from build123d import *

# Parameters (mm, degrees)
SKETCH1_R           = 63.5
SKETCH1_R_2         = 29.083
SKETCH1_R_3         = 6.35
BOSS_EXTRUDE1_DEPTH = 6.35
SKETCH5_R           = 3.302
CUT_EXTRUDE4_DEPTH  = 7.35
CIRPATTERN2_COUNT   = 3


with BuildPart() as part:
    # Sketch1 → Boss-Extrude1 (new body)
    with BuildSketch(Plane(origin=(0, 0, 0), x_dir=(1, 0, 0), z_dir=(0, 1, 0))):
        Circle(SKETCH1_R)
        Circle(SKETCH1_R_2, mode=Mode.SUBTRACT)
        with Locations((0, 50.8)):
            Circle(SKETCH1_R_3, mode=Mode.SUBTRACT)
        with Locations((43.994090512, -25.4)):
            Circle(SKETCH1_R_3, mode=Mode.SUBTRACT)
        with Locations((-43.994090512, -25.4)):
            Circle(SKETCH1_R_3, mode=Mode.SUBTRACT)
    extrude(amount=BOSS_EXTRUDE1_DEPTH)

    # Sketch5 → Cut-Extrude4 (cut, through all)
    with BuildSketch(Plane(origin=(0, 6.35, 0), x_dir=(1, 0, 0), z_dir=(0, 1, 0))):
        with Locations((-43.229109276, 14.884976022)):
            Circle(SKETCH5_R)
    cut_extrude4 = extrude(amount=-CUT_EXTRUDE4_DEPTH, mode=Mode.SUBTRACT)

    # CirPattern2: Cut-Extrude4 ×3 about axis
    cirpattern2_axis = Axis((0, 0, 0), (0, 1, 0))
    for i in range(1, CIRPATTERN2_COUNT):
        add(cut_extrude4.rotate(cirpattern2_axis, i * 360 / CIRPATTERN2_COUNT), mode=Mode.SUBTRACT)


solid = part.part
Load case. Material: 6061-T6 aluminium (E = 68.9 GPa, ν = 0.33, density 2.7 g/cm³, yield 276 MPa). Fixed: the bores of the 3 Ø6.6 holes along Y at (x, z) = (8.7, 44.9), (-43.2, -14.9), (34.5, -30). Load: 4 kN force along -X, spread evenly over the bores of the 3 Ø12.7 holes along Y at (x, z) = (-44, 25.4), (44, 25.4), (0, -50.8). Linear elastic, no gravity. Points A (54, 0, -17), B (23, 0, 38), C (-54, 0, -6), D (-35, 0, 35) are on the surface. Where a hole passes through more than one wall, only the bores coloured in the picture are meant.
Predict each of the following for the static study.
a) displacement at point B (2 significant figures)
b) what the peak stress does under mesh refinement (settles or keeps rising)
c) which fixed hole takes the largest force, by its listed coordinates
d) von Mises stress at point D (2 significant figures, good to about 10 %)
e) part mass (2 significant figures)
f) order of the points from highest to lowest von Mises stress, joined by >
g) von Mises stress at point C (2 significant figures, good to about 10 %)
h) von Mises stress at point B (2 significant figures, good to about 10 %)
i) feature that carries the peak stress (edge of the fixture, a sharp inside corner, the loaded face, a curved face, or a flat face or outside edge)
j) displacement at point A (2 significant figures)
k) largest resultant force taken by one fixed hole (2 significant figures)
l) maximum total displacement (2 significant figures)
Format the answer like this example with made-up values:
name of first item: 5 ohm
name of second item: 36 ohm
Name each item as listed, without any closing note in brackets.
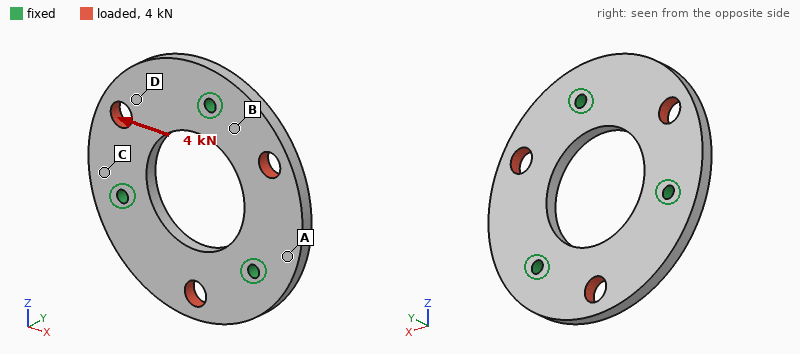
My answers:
displacement at point B: 2.6 µm
what the peak stress does under mesh refinement: keeps rising
which fixed hole takes the largest force, by its listed coordinates: (8.7, 44.9)
von Mises stress at point D: 6.7 MPa
part mass: 160 g
order of the points from highest to lowest von Mises stress, joined by >: B > D > C > A
von Mises stress at point C: 3.7 MPa
von Mises stress at point B: 8.3 MPa
feature that carries the peak stress: edge of the fixture
displacement at point A: 1.4 µm
largest resultant force taken by one fixed hole: 2.0 kN
maximum total displacement: 7.3 µm
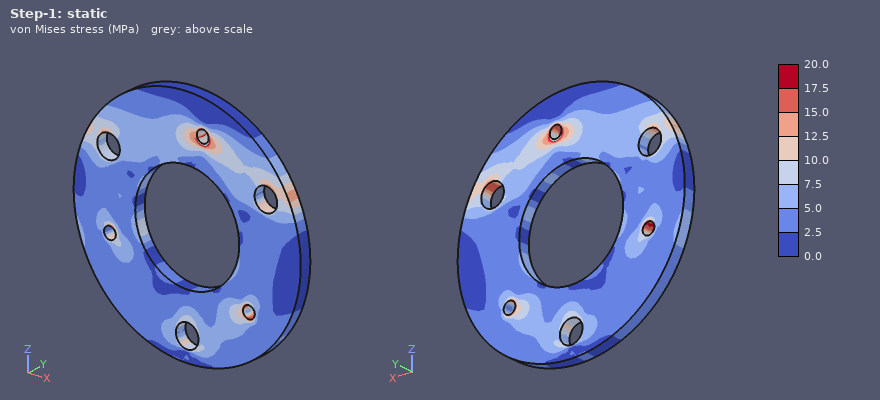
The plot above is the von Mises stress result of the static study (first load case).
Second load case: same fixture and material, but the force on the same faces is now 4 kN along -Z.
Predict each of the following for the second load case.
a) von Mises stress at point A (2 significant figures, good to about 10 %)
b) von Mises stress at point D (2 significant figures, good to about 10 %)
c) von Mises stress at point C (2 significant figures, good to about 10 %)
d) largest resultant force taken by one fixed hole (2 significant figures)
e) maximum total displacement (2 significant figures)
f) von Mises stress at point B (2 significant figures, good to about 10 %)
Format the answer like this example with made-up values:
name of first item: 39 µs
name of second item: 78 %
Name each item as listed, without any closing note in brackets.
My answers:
von Mises stress at point A: 3.5 MPa
von Mises stress at point D: 3.0 MPa
von Mises stress at point C: 5.0 MPa
largest resultant force taken by one fixed hole: 1.8 kN
maximum total displacement: 7.5 µm
von Mises stress at point B: 4.0 MPa
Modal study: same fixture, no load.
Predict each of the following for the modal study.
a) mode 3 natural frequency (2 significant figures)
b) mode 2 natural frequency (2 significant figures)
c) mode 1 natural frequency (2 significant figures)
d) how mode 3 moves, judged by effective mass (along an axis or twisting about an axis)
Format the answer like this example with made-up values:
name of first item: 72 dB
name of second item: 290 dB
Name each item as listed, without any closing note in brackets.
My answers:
mode 3 natural frequency: 2900 Hz
mode 2 natural frequency: 2700 Hz
mode 1 natural frequency: 2700 Hz
how mode 3 moves, judged by effective mass: along Y
